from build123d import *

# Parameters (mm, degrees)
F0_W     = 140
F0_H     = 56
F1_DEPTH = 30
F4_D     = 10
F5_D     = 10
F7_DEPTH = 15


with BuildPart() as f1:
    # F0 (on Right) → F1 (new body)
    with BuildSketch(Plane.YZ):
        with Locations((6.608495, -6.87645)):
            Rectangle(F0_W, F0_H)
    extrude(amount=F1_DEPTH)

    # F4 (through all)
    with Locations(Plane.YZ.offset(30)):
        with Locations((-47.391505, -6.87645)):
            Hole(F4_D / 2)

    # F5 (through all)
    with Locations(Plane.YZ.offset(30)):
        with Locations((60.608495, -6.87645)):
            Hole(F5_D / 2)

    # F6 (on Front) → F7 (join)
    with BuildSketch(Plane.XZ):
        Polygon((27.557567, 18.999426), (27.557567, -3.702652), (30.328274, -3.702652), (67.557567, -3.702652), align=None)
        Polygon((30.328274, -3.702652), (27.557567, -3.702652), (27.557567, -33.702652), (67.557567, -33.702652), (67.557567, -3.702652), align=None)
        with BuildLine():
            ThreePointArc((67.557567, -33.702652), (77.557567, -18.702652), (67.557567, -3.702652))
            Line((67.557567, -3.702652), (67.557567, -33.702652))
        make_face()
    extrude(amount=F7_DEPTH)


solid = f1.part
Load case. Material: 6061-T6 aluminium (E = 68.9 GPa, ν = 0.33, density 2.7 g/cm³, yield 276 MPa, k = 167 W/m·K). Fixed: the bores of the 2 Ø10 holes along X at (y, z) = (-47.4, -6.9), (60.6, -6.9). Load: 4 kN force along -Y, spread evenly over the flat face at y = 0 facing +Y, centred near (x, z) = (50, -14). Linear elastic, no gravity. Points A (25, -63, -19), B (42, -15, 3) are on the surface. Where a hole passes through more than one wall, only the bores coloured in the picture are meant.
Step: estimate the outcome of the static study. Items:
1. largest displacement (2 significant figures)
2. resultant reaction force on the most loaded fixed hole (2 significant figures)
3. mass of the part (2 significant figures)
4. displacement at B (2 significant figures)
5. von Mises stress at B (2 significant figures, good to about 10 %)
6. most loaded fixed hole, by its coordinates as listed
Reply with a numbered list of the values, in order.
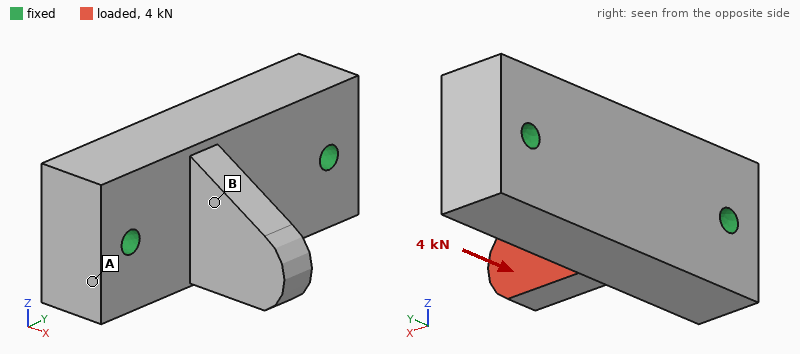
1. 87 µm
2. 2.8 kN
3. 690 g
4. 17 µm
5. 25 MPa
6. (-47.4, -6.9)
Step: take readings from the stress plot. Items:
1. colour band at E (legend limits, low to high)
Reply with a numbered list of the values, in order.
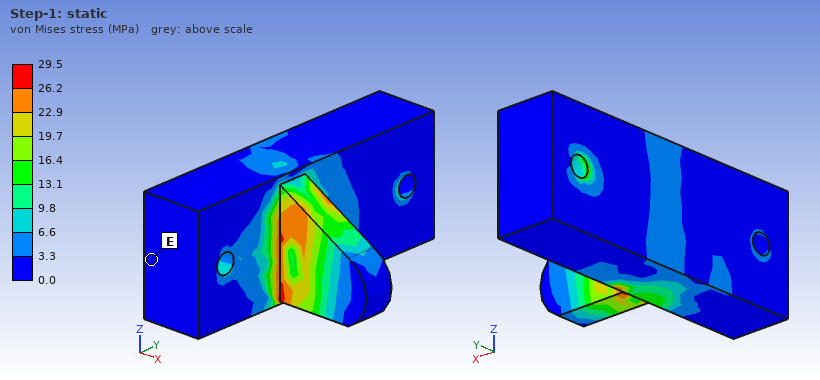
1. 0.0 to 3.3 MPa
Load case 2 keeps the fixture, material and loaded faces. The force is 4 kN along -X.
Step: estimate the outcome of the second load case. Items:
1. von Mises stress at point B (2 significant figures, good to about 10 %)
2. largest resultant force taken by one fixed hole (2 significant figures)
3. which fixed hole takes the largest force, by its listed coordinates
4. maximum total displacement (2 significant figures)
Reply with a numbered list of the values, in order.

1. 9.2 MPa
2. 2.3 kN
3. (-47.4, -6.9)
4. 41 µm
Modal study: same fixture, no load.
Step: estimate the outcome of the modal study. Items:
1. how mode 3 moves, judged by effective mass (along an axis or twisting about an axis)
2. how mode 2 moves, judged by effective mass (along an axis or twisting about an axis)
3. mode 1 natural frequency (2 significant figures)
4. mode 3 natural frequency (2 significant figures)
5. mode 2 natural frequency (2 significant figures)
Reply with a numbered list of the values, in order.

1. along X
2. along Z
3. 5200 Hz
4. 7500 Hz
5. 5900 Hz
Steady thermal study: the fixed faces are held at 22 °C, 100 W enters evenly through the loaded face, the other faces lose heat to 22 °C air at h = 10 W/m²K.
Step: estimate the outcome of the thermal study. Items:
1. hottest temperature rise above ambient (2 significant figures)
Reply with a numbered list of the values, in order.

1. 35 K
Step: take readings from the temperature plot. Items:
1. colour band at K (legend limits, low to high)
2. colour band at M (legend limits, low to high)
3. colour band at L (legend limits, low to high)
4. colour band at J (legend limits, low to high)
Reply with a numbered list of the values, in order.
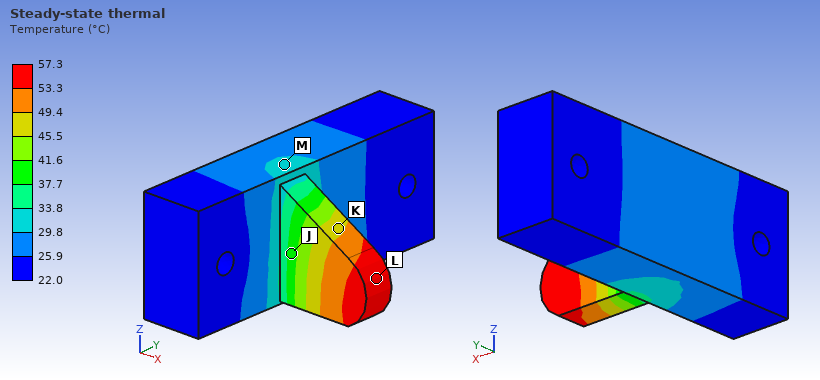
1. 45.5 to 49.4 °C
2. 29.8 to 33.8 °C
3. 53.3 to 57.3 °C
4. 37.7 to 41.6 °C
